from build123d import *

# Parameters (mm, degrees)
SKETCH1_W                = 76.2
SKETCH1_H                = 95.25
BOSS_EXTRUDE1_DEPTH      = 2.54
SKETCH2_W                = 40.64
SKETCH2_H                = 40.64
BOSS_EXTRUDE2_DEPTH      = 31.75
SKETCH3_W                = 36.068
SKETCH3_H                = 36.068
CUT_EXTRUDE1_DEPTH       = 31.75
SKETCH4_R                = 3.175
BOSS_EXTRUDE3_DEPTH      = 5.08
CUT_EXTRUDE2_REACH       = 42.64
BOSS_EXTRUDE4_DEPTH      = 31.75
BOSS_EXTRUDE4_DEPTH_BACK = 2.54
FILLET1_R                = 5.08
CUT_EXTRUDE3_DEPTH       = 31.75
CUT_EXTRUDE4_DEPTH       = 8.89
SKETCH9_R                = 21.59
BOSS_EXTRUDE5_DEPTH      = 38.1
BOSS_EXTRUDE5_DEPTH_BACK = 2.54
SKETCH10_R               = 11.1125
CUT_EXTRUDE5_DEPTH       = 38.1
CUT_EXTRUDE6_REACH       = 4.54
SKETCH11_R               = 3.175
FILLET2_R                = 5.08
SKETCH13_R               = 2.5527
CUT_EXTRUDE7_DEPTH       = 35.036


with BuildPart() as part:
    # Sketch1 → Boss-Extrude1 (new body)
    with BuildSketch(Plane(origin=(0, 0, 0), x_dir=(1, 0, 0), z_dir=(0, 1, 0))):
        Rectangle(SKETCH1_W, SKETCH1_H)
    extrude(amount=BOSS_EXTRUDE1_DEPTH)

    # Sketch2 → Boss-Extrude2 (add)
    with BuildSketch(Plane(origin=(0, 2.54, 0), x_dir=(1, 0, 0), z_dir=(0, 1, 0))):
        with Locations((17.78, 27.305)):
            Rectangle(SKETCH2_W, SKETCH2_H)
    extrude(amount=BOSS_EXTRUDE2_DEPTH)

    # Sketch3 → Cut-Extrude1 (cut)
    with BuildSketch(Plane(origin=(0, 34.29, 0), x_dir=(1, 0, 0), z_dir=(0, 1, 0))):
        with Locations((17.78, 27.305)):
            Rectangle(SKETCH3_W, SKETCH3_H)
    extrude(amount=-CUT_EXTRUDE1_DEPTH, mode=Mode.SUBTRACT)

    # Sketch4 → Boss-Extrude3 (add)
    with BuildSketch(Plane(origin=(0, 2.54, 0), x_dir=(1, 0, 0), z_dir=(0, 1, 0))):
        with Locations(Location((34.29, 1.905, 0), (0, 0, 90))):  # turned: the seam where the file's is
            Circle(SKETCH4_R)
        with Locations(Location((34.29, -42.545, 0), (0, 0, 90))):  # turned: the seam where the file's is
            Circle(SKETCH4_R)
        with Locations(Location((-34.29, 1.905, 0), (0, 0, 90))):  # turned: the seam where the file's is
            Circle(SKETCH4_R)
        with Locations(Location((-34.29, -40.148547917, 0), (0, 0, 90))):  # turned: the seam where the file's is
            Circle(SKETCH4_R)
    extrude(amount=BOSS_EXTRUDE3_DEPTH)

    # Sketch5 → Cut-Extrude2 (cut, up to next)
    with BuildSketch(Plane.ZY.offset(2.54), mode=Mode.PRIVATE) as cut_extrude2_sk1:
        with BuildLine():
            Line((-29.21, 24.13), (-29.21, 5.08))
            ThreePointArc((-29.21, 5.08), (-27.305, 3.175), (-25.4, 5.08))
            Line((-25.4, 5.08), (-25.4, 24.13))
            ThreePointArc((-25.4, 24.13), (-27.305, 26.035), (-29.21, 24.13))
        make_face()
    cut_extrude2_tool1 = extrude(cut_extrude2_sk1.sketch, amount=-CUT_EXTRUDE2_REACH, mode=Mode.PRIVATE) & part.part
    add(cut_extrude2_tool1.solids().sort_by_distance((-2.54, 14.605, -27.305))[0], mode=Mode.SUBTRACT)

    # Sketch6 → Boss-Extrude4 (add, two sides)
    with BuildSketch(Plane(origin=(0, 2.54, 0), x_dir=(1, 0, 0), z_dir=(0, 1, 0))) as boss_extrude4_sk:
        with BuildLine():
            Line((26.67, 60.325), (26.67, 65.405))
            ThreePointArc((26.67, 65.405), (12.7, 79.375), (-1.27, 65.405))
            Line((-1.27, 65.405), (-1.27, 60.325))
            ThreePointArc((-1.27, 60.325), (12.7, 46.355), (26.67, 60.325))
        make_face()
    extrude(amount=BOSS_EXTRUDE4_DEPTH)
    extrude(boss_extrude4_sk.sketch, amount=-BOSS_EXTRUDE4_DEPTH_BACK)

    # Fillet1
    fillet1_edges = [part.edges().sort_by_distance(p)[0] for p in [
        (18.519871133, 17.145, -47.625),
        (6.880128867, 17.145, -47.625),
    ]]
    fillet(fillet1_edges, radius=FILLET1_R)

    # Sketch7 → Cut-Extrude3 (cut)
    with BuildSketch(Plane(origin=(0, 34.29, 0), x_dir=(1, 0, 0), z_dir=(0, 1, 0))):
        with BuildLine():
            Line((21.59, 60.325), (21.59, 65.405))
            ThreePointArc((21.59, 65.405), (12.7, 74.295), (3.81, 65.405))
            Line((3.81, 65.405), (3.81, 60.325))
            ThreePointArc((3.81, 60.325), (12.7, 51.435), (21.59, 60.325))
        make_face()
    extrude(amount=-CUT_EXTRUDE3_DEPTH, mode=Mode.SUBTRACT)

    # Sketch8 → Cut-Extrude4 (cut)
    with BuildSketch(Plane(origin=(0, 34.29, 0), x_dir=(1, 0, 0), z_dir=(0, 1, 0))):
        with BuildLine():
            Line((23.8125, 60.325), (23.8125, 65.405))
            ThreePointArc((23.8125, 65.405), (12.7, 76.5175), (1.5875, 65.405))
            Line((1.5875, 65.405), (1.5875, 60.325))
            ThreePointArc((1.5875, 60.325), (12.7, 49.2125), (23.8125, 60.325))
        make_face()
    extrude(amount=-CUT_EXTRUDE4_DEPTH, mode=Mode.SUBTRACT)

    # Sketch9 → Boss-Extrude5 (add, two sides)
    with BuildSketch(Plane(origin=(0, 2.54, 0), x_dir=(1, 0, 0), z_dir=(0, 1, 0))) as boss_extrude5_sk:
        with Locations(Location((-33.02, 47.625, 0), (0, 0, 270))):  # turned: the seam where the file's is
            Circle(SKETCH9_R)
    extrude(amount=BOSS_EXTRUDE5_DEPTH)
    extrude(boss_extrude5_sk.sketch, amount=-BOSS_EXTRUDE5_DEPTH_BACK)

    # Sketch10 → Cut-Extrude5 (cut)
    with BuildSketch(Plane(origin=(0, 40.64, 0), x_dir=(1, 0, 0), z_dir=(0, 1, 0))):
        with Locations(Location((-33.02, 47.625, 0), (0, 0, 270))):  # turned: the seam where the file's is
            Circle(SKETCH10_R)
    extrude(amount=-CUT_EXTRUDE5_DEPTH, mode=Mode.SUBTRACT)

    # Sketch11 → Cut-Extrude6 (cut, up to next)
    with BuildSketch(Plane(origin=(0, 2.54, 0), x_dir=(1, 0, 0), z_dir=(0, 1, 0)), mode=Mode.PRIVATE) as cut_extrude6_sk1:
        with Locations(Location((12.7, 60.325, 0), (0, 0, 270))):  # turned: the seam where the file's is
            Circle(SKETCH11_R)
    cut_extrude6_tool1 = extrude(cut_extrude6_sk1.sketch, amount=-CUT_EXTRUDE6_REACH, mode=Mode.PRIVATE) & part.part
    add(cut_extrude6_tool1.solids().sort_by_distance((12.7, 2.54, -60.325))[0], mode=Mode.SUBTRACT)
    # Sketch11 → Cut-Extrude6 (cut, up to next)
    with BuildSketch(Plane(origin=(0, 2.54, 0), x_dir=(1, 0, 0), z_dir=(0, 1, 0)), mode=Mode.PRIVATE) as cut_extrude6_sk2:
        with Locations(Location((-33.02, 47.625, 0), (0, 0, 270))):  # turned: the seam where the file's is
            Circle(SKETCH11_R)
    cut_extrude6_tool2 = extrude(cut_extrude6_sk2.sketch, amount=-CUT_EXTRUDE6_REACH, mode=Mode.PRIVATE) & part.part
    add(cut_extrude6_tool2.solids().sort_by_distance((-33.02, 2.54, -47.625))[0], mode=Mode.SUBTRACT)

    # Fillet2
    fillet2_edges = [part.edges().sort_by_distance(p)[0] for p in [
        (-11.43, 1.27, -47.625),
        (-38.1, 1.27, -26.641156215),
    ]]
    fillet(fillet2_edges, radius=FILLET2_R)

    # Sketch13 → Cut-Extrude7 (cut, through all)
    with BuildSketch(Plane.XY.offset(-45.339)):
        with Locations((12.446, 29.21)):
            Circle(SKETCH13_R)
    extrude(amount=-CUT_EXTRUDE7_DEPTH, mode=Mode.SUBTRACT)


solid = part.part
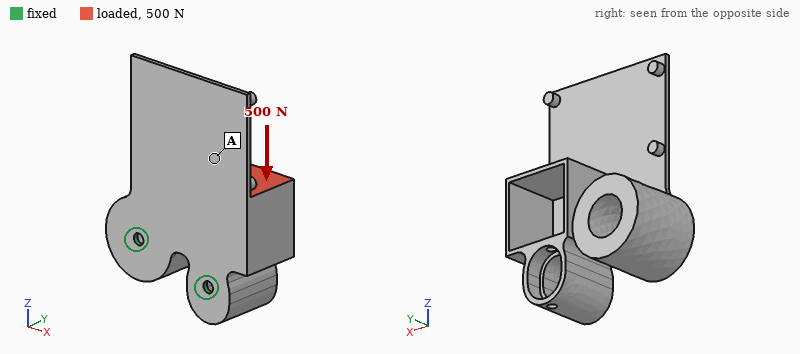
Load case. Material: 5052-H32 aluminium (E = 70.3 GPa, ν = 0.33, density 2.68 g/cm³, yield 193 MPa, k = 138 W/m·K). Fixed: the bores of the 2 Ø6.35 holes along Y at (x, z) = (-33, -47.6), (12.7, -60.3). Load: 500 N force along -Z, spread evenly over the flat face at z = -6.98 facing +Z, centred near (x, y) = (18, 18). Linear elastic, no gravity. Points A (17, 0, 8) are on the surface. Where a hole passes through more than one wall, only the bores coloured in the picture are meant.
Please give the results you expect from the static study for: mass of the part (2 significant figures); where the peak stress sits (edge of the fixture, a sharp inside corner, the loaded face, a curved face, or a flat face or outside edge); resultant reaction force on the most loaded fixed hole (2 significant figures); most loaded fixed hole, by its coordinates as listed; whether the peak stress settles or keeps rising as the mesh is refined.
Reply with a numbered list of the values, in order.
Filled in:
1. 240 g
2. edge of the fixture
3. 530 N
4. (12.7, -60.3)
5. keeps rising
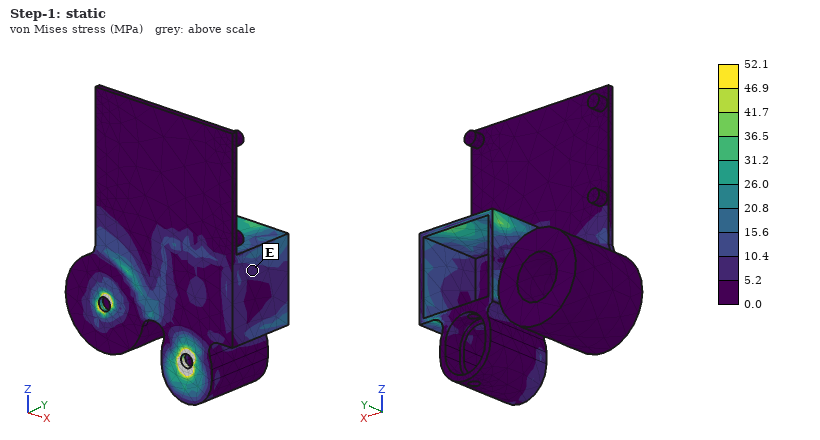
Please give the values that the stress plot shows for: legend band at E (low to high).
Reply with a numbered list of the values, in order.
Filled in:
1. 5.2 to 10.4 MPa
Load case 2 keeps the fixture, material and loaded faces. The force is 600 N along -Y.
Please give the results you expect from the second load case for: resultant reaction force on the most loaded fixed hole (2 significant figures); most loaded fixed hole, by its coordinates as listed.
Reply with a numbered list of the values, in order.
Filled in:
1. 360 N
2. (12.7, -60.3)
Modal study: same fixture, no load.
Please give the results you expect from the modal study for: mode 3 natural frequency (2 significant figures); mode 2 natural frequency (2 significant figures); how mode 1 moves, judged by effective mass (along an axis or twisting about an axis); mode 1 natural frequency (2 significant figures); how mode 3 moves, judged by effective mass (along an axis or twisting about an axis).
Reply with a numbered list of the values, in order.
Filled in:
1. 940 Hz
2. 840 Hz
3. along Y
4. 420 Hz
5. along Z
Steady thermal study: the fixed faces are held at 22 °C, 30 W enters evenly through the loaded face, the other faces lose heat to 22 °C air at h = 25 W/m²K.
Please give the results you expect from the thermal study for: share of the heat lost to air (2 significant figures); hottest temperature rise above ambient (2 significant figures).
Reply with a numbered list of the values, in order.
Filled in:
1. 43 %
2. 45 K
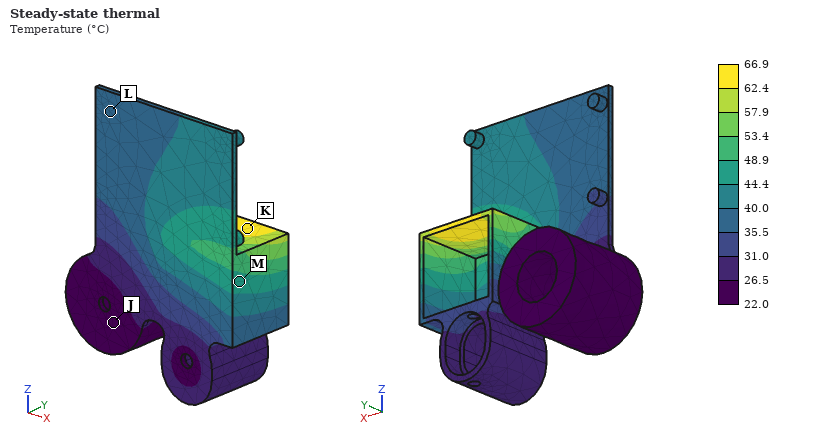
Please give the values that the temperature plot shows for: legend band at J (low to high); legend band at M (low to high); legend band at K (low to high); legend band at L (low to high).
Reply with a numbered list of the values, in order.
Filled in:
1. 22.0 to 26.5 °C
2. 44.4 to 48.9 °C
3. 62.4 to 66.9 °C
4. 35.5 to 40.0 °C
